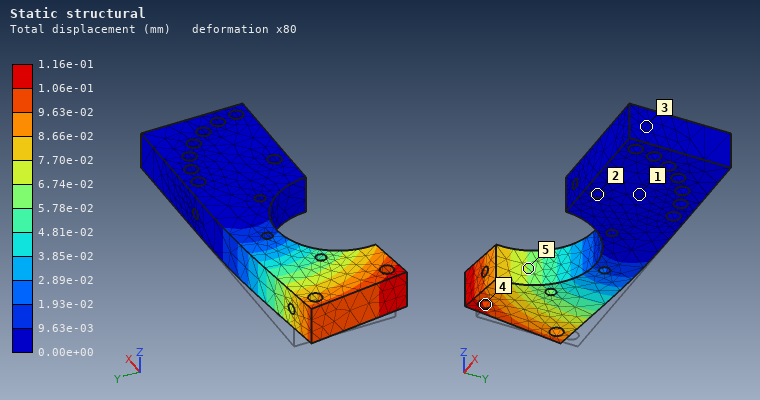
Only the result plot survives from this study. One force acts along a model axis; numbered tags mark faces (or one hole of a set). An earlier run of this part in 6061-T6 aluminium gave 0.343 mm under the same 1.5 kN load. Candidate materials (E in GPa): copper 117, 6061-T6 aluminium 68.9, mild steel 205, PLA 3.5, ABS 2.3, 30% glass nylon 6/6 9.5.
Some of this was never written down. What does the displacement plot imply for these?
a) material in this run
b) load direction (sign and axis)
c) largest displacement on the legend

mild steel
-Y
1.16e-01 mm
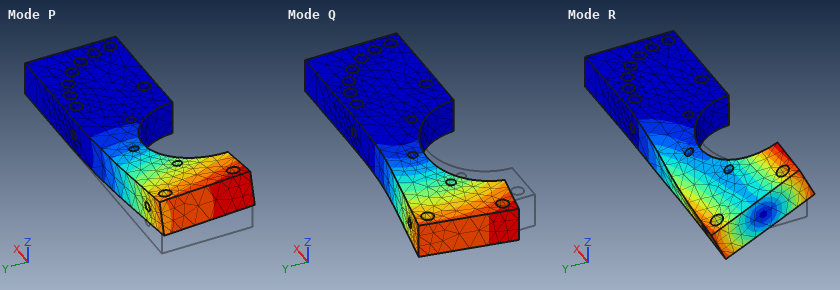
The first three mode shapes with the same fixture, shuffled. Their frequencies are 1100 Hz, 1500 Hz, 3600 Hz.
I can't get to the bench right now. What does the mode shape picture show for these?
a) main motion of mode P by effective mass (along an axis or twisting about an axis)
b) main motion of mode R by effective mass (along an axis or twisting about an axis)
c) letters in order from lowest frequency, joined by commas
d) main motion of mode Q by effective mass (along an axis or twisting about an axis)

along Z
twisting about X
P, Q, R
along Y
